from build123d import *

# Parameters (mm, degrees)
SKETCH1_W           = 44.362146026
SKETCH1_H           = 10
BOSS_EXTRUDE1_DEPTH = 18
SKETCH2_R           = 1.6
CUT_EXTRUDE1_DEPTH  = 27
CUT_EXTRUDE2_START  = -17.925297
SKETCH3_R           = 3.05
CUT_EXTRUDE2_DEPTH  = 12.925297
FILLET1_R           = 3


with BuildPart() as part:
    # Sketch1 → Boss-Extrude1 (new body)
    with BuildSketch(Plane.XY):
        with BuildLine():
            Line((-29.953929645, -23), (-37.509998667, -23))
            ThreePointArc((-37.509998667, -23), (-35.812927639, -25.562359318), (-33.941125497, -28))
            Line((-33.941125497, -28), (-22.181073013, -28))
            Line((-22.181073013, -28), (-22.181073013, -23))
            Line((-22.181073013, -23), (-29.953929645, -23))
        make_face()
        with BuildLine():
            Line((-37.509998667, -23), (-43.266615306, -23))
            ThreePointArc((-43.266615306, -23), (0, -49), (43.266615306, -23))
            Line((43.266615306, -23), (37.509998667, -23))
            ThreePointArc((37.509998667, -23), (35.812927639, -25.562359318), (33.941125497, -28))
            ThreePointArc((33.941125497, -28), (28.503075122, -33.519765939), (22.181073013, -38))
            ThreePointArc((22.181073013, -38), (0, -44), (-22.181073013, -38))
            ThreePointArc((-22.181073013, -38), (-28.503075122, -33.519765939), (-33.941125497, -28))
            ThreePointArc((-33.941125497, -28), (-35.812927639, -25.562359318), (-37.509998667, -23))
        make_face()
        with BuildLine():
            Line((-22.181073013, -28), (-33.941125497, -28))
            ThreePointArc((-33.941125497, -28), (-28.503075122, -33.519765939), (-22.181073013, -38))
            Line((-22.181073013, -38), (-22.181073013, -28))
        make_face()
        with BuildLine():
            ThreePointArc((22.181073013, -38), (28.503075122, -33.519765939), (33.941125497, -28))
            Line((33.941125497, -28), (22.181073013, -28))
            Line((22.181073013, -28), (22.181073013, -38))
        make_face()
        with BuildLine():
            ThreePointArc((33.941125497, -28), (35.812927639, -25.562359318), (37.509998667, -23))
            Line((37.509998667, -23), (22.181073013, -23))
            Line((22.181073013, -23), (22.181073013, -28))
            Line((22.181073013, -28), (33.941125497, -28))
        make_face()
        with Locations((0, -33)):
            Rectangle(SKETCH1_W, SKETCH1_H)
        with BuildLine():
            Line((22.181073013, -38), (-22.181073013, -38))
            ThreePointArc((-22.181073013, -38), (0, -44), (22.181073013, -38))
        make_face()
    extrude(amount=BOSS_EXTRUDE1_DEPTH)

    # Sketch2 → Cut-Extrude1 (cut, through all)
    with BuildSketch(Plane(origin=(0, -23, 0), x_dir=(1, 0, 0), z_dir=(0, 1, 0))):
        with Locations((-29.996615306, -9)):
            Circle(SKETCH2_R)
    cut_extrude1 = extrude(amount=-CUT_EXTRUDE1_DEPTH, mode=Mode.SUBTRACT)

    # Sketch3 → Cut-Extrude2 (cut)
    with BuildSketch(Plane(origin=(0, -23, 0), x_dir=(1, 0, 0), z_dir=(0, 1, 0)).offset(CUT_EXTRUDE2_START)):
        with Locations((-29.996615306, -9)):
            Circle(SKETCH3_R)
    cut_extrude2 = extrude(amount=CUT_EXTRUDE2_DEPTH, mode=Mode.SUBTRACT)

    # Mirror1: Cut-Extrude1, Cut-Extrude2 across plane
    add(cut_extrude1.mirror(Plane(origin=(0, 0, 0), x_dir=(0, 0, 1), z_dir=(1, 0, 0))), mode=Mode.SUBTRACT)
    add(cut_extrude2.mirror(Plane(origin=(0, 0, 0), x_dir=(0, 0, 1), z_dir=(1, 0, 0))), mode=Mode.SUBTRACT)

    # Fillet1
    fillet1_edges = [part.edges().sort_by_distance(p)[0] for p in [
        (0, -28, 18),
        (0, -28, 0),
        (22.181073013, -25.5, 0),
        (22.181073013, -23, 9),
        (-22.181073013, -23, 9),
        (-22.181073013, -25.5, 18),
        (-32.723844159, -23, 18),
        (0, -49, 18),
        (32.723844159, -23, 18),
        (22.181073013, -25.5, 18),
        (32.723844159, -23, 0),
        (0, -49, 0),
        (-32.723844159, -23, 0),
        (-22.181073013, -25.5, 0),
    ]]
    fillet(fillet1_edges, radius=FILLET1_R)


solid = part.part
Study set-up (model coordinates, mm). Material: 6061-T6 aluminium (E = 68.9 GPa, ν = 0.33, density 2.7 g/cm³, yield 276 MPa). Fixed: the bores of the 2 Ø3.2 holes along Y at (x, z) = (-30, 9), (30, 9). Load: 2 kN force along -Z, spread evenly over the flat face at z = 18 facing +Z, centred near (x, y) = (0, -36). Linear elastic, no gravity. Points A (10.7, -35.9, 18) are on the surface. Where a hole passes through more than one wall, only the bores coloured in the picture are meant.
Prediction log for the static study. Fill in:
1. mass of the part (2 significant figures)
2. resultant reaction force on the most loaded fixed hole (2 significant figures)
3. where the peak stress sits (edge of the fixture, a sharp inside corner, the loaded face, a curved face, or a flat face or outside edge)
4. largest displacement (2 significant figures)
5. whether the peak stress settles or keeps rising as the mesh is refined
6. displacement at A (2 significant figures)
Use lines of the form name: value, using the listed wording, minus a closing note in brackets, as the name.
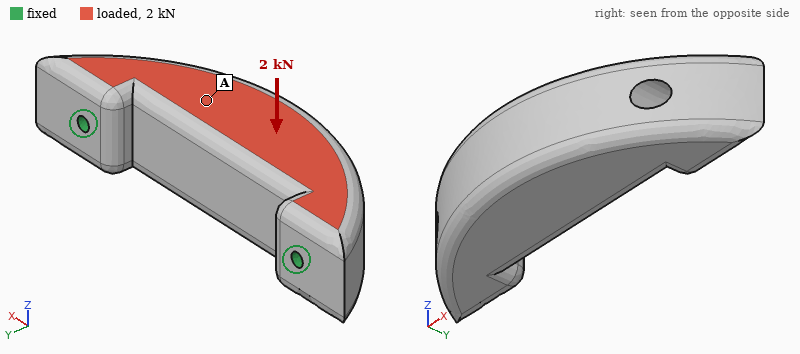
mass of the part: 63 g
resultant reaction force on the most loaded fixed hole: 1.0 kN
where the peak stress sits: edge of the fixture
largest displacement: 66 µm
whether the peak stress settles or keeps rising as the mesh is refined: keeps rising
displacement at A: 39 µm
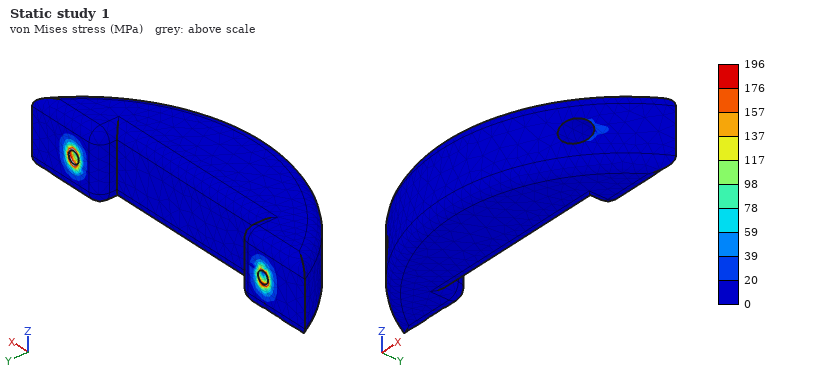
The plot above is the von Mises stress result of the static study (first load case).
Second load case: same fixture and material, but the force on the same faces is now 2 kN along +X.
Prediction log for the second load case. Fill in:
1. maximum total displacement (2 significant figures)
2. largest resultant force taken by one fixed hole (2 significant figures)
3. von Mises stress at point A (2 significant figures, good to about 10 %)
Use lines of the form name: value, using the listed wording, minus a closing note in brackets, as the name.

maximum total displacement: 6.1 µm
largest resultant force taken by one fixed hole: 1.1 kN
von Mises stress at point A: 8.1 MPa
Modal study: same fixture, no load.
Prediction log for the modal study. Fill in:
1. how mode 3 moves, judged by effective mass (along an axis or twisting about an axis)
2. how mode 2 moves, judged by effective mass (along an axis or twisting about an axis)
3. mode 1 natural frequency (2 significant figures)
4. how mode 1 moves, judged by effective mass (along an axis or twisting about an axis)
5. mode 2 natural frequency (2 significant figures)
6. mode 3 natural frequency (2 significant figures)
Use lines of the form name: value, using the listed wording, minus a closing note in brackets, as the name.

how mode 3 moves, judged by effective mass: along X
how mode 2 moves, judged by effective mass: along Y
mode 1 natural frequency: 4500 Hz
how mode 1 moves, judged by effective mass: along Z
mode 2 natural frequency: 13 kHz
mode 3 natural frequency: 15 kHz
